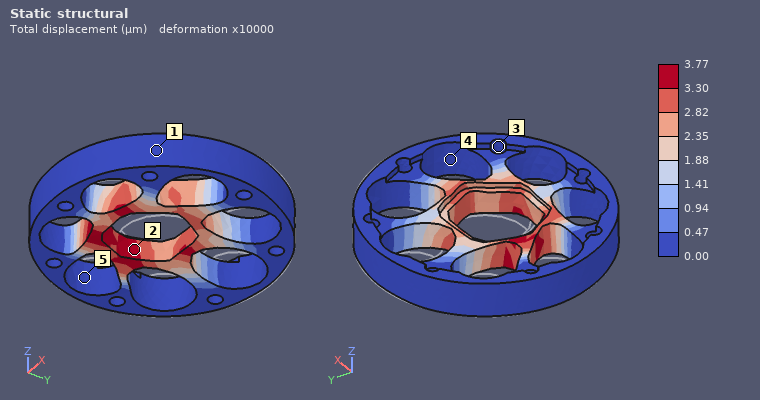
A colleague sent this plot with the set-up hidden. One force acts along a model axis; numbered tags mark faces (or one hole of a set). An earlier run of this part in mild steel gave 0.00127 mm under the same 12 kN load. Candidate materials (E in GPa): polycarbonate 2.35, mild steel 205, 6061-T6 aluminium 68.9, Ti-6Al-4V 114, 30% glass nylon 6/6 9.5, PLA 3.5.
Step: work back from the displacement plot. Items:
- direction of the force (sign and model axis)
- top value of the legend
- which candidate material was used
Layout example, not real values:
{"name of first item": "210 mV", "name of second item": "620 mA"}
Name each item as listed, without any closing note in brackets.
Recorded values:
{"direction of the force": "-Y", "top value of the legend": "3.77 µm", "which candidate material was used": "6061-T6 aluminium"}
